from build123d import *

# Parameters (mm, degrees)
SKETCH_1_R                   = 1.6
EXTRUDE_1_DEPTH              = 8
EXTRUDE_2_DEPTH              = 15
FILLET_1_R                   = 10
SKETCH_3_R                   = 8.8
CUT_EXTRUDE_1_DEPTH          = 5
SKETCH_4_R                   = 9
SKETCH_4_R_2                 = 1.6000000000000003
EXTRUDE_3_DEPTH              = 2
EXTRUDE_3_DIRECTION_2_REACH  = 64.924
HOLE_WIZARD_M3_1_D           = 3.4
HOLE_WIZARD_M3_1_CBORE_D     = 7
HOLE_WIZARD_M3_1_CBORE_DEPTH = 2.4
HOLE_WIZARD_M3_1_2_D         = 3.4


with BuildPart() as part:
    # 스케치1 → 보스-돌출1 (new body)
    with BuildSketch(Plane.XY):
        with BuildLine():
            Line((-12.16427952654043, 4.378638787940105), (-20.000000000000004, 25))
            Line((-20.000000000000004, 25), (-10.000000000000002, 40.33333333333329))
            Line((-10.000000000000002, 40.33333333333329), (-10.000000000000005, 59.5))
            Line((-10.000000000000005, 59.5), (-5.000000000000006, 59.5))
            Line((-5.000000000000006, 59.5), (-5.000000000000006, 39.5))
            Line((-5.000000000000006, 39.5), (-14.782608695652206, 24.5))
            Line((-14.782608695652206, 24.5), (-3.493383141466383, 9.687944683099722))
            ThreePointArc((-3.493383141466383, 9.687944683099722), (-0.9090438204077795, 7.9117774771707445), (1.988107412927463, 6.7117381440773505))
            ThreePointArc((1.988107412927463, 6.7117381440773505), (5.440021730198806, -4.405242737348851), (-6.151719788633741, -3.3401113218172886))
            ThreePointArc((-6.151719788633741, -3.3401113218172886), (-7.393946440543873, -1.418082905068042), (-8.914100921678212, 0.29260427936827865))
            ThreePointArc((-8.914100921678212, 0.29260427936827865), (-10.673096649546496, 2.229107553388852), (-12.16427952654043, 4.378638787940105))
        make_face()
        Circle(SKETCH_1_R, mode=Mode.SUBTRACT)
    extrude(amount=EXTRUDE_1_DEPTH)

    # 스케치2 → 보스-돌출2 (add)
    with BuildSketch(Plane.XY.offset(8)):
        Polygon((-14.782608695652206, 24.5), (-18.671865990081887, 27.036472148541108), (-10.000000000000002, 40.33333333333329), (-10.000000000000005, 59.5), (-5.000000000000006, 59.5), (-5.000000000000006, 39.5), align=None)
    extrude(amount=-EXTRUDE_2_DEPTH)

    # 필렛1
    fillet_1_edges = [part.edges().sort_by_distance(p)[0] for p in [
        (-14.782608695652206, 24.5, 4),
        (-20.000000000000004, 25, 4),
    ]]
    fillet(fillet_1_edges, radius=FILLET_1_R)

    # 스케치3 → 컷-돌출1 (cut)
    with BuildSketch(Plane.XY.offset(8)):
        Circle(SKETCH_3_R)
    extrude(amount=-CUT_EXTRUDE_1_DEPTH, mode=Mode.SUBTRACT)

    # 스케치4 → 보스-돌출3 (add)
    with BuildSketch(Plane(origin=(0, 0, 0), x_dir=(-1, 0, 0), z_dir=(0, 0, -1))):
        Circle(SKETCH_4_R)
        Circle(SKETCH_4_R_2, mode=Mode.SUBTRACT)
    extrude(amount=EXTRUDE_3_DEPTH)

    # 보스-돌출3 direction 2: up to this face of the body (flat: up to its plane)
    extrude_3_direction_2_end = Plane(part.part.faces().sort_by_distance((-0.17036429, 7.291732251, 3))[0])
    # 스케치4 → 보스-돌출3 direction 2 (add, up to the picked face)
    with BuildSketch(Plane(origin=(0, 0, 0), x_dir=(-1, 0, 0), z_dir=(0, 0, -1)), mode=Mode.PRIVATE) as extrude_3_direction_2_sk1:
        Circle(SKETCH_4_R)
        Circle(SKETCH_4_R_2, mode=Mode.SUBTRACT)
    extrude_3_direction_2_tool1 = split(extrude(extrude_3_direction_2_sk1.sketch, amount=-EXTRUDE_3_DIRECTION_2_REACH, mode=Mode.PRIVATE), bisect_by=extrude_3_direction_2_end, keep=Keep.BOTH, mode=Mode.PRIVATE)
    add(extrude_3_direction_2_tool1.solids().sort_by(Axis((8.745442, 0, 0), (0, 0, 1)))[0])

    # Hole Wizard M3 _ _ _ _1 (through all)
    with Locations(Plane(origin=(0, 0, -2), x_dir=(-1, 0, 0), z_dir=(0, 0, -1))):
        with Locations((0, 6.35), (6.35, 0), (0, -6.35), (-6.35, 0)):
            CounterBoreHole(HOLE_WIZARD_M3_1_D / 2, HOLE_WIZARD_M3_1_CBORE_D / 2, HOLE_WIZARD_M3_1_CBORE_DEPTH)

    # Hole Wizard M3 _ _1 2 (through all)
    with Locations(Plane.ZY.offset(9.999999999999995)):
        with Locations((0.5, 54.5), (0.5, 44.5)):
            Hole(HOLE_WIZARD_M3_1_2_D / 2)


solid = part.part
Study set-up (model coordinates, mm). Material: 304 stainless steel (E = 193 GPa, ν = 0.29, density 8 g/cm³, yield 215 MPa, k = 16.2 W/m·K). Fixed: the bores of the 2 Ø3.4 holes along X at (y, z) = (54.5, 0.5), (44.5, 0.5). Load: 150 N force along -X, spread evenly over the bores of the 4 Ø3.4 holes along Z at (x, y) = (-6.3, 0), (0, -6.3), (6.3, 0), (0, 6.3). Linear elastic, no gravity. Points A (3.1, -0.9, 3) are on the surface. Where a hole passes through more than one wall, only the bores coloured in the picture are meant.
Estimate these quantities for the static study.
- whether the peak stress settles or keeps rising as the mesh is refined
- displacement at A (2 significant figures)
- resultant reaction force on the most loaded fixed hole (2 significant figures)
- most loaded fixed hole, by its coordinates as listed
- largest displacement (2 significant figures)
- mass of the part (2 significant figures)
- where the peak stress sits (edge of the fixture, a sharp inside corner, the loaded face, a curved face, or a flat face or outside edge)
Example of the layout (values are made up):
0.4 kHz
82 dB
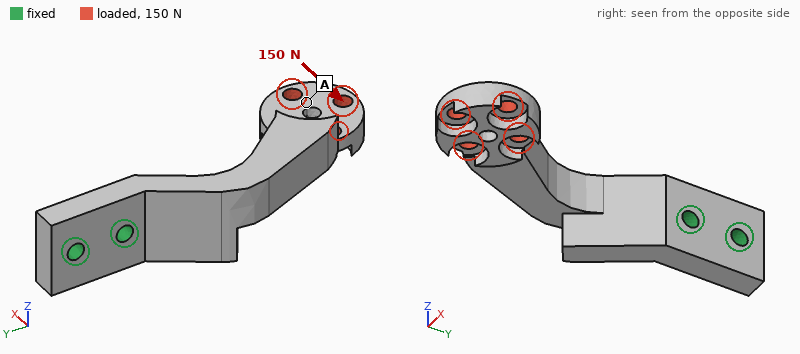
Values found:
keeps rising
0.20 mm
340 N
(44.5, 0.5)
0.25 mm
38 g
edge of the fixture
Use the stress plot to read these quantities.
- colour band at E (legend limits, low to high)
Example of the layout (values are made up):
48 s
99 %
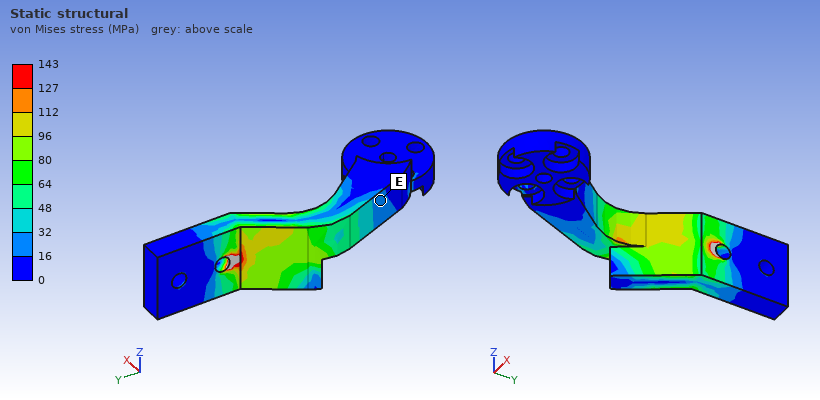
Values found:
16 to 32 MPa
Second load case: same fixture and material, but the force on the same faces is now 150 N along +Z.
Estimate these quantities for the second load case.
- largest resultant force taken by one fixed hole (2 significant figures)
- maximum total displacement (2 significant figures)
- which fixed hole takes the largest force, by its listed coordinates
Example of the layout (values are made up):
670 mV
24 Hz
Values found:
550 N
0.16 mm
(44.5, 0.5)
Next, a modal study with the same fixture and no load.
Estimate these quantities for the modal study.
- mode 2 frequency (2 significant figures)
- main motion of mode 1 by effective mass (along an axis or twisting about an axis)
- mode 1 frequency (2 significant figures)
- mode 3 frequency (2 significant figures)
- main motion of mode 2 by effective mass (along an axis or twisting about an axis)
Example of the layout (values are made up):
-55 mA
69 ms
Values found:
2000 Hz
along X
1300 Hz
5700 Hz
along Z
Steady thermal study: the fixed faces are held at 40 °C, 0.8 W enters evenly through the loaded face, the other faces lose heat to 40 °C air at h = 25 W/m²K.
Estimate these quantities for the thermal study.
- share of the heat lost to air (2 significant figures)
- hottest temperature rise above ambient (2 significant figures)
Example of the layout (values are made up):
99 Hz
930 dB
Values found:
73 %
20 K
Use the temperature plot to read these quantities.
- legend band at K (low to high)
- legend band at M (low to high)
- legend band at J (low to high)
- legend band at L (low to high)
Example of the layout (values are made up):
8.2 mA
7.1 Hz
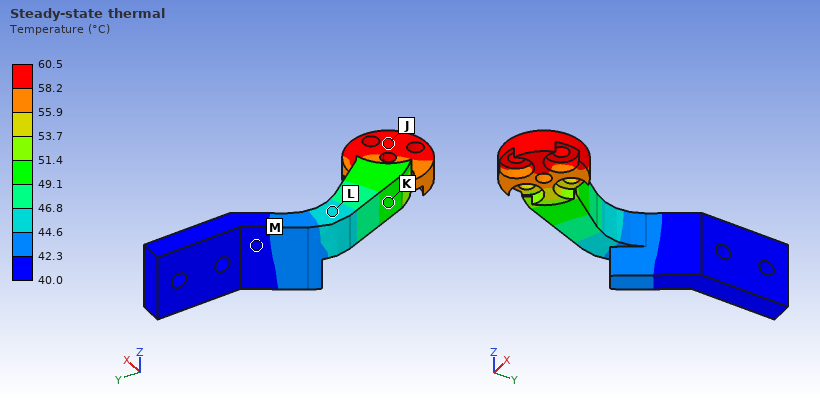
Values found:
49.1 to 51.4 °C
40.0 to 42.3 °C
58.2 to 60.5 °C
44.6 to 46.8 °C
